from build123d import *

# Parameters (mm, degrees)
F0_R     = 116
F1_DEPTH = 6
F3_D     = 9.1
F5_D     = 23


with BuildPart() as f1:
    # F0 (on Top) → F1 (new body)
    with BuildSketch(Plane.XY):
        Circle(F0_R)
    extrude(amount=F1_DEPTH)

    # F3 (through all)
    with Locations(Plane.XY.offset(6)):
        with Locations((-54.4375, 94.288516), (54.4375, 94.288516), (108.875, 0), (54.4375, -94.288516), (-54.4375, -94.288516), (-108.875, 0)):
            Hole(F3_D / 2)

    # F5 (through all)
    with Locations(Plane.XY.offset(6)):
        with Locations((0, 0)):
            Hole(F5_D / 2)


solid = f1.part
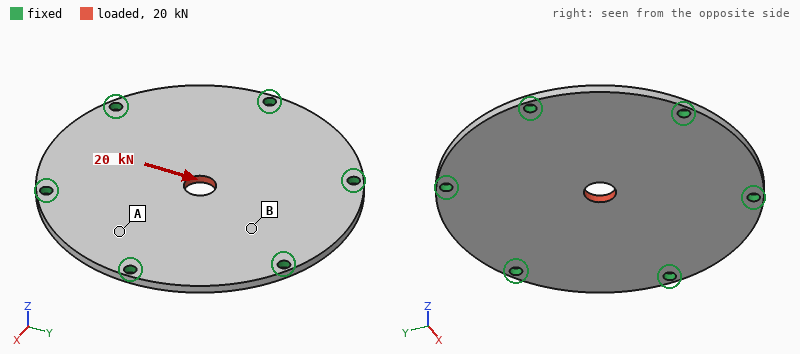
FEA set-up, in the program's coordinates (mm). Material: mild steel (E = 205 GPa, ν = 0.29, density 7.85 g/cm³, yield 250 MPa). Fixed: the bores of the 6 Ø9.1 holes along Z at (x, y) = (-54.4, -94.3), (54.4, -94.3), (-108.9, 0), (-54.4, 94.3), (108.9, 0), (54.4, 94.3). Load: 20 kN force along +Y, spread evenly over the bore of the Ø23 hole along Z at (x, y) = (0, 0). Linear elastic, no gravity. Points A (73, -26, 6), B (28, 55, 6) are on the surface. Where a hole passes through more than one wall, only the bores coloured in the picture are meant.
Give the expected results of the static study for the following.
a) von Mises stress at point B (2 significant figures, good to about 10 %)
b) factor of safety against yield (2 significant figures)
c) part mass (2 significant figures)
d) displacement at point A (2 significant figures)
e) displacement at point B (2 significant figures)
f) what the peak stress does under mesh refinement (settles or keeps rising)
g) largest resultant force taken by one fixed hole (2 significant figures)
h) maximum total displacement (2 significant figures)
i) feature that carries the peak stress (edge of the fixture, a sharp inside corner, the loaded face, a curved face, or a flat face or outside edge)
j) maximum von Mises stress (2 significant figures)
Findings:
18 MPa
3.1
2.0 kg
3.0 µm
5.2 µm
settles
4.3 kN
12 µm
the loaded face
80 MPa
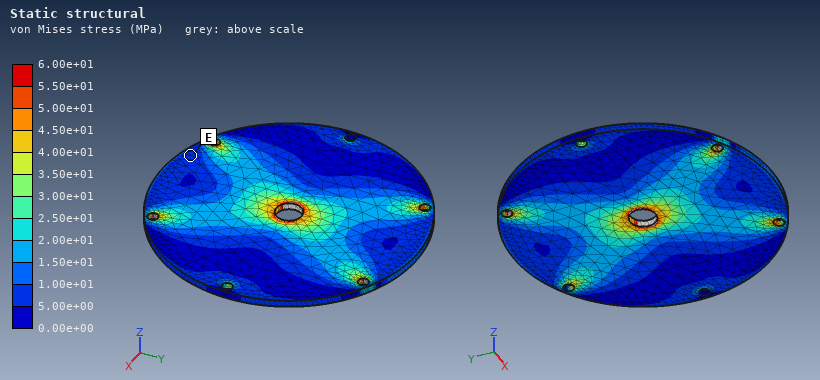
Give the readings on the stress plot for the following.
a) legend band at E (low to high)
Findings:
5.00e+00 to 1.00e+01 MPa
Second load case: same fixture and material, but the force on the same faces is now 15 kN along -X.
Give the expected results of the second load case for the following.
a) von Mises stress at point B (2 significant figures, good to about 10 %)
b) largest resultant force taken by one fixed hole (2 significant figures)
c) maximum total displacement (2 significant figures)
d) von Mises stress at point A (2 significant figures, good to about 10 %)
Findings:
8.1 MPa
3.7 kN
9.3 µm
8.1 MPa
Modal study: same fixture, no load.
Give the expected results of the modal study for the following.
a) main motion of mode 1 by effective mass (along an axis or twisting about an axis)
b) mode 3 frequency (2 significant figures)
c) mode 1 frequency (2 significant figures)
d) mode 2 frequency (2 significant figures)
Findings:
along Z
2100 Hz
1000 Hz
2100 Hz
